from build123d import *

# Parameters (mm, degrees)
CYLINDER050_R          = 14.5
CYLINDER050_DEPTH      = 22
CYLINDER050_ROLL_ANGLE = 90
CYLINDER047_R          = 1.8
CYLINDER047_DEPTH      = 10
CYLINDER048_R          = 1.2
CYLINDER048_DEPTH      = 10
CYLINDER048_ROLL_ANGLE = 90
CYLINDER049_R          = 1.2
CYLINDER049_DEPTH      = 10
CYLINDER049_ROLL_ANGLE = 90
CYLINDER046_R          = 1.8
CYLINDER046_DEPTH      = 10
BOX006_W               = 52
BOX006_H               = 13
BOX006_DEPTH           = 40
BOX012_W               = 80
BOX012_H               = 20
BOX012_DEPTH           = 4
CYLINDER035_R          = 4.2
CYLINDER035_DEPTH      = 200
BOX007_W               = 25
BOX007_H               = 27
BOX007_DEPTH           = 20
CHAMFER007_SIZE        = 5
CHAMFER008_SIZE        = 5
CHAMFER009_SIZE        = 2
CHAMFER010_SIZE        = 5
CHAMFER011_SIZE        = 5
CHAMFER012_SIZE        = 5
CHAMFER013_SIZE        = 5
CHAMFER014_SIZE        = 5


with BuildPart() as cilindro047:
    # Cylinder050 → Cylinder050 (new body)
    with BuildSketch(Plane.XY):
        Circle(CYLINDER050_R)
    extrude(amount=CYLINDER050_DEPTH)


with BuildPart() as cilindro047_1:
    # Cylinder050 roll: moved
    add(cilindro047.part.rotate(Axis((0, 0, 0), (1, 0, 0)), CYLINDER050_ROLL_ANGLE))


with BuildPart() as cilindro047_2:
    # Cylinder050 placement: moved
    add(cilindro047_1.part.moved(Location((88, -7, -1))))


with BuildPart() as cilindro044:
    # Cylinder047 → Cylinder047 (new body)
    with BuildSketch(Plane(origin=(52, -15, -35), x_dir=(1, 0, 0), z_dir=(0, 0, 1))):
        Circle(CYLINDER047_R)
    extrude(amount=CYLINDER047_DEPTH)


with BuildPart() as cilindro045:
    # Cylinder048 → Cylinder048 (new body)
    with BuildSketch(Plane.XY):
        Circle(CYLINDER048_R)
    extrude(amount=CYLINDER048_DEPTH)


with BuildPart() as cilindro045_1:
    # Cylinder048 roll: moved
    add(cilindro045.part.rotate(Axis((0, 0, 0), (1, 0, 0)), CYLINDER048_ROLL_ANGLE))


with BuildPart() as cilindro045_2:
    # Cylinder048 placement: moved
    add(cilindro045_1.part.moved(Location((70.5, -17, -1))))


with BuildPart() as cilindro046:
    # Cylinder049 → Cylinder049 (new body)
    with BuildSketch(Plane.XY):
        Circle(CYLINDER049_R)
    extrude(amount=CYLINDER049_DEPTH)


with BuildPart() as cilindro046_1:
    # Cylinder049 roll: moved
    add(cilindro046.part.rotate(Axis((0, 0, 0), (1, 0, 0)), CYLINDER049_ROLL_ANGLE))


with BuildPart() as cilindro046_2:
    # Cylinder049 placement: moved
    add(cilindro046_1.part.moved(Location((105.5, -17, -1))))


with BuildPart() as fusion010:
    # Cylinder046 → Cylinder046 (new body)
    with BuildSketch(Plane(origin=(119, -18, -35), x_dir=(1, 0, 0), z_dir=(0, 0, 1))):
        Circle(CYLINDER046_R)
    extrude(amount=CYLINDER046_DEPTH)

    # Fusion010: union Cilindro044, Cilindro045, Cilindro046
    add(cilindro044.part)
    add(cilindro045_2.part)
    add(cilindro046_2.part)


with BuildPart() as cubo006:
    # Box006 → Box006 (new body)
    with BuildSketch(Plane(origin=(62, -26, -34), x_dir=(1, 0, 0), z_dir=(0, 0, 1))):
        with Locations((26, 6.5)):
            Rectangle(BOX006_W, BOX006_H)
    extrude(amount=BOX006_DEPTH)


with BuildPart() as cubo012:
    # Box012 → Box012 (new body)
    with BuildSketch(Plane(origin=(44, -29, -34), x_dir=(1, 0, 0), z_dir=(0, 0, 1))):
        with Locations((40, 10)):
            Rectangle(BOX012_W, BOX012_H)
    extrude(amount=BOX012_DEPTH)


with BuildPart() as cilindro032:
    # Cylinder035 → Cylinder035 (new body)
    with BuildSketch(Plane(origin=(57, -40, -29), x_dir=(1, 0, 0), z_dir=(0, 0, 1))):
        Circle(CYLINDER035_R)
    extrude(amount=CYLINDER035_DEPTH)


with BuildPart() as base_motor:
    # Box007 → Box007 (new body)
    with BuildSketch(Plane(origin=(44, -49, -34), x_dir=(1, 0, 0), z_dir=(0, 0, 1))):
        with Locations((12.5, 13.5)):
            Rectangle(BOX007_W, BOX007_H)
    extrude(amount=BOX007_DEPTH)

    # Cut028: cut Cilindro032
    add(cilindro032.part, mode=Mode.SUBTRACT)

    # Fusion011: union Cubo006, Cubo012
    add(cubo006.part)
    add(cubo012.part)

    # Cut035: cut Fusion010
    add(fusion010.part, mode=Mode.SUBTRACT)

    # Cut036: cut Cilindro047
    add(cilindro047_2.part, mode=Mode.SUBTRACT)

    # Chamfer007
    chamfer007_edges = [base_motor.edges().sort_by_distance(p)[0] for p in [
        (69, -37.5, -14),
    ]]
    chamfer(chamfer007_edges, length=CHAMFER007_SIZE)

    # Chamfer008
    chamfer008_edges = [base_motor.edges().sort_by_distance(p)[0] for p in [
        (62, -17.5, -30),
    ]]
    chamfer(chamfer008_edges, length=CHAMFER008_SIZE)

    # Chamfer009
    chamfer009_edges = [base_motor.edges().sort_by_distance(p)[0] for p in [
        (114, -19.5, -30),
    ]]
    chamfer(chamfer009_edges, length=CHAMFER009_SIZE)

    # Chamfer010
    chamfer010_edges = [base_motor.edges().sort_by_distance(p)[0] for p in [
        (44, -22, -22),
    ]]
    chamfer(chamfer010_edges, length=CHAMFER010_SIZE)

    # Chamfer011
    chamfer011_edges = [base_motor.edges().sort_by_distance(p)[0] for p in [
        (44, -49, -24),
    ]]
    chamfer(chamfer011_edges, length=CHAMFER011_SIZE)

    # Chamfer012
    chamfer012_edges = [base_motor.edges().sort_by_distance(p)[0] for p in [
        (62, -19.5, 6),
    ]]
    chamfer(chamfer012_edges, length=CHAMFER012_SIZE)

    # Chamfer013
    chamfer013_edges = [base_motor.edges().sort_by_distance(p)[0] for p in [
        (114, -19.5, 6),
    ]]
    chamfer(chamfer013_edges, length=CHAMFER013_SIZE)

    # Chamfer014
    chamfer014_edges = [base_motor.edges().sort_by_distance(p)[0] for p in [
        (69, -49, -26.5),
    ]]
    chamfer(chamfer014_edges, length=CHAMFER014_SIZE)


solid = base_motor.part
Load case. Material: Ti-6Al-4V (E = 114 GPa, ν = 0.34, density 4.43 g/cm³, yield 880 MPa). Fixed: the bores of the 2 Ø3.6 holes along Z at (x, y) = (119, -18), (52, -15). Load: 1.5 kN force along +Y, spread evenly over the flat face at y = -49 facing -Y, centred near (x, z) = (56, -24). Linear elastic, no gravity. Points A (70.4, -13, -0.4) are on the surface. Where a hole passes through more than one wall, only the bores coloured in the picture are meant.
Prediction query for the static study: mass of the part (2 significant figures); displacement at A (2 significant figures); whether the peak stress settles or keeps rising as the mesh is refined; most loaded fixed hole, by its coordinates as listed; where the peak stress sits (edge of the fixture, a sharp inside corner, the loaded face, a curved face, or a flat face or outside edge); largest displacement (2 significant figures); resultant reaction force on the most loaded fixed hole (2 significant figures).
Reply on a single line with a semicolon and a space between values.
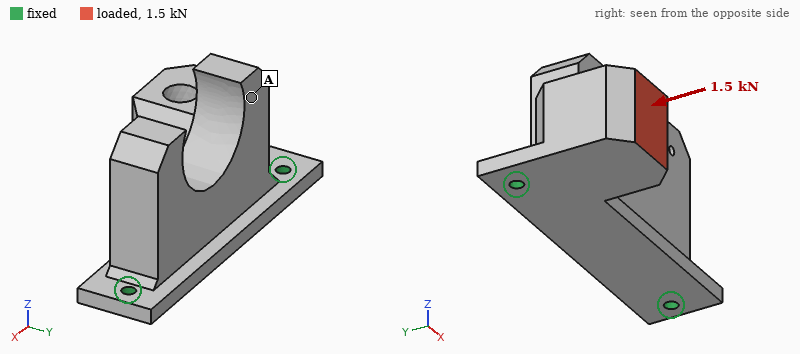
150 g; 0.083 mm; keeps rising; (52, -15); edge of the fixture; 0.10 mm; 1.4 kN
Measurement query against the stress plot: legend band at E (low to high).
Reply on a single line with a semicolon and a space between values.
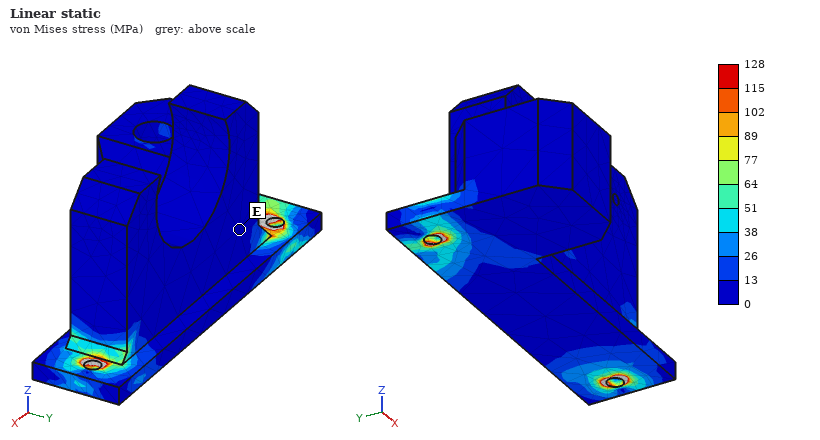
0 to 13 MPa
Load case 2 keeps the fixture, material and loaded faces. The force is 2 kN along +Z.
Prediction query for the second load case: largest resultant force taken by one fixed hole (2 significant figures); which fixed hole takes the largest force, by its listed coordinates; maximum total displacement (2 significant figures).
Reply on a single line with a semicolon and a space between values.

1.8 kN; (52, -15); 0.54 mm
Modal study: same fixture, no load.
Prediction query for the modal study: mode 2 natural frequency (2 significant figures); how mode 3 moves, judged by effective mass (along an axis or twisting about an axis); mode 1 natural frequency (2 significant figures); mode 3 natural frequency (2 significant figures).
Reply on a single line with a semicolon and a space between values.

4900 Hz; along X; 1500 Hz; 6200 Hz
